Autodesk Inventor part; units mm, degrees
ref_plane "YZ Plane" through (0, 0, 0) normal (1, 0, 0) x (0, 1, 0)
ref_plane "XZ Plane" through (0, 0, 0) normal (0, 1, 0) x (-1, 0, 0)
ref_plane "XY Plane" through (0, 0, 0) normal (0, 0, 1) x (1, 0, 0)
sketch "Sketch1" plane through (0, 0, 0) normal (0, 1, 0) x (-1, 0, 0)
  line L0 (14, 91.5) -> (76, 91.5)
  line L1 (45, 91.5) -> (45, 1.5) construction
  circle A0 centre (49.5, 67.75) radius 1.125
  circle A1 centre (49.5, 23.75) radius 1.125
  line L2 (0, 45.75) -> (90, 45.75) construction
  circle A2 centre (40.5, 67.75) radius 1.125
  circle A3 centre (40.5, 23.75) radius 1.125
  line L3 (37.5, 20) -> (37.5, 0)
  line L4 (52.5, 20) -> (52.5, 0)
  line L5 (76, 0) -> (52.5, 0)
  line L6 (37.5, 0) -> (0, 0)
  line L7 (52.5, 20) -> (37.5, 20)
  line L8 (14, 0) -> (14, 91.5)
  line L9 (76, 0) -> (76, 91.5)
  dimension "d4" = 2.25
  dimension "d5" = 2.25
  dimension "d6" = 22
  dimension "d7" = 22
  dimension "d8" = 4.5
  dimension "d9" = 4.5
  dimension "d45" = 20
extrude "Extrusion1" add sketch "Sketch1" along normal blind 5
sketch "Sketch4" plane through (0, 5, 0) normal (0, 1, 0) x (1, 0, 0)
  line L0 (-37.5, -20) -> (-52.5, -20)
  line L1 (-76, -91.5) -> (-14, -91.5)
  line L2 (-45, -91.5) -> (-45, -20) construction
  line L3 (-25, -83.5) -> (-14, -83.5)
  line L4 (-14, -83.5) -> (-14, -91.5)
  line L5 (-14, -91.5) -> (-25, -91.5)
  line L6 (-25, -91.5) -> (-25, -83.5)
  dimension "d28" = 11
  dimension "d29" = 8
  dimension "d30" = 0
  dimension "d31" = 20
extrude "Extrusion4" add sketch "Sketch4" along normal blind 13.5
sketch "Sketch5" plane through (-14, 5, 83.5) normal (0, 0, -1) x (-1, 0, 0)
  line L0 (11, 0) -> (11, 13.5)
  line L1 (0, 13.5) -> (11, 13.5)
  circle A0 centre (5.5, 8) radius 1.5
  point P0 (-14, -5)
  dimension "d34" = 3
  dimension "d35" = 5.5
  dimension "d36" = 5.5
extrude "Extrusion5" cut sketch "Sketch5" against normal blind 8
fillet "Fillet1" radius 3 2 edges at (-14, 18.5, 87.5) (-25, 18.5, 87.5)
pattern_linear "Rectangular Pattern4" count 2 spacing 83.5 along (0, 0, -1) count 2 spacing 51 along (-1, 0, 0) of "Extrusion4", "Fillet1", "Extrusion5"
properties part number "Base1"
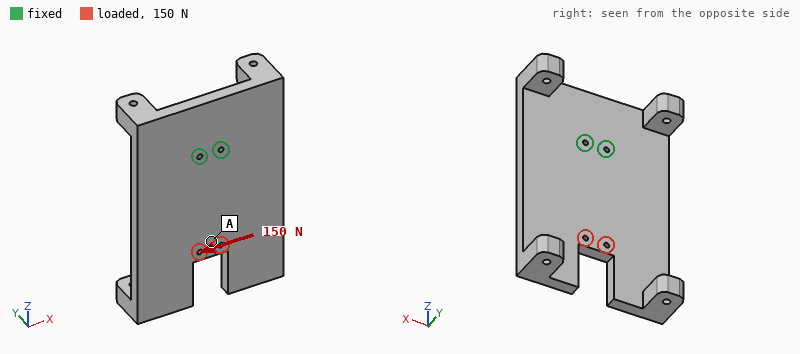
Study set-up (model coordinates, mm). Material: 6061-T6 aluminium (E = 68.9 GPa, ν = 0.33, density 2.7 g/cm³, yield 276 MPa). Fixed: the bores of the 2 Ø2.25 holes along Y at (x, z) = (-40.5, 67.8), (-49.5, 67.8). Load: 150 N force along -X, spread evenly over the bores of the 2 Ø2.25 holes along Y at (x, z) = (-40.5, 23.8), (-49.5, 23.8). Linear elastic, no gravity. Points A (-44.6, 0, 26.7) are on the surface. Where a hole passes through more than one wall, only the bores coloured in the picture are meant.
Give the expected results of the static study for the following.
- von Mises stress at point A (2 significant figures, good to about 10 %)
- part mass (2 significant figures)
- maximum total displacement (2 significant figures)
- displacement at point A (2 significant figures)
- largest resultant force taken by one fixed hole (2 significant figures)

1.8 MPa
84 g
21 µm
12 µm
630 N
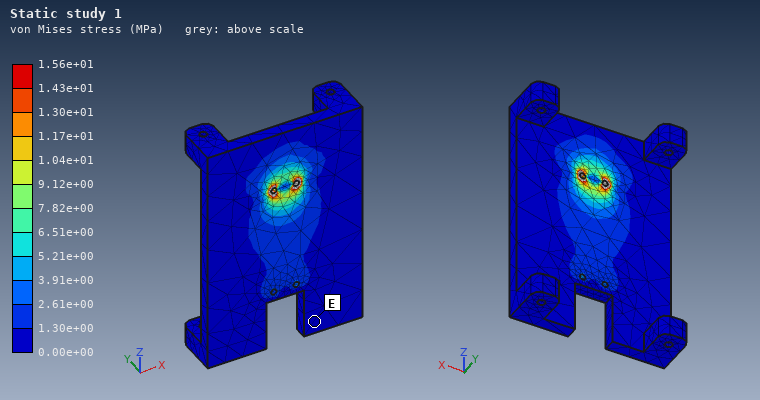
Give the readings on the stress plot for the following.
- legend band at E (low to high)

0.00e+00 to 1.30e+00 MPa
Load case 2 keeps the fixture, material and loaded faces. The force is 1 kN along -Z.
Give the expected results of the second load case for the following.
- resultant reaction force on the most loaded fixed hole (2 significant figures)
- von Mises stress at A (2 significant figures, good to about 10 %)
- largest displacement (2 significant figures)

500 N
6.9 MPa
5.5 µm
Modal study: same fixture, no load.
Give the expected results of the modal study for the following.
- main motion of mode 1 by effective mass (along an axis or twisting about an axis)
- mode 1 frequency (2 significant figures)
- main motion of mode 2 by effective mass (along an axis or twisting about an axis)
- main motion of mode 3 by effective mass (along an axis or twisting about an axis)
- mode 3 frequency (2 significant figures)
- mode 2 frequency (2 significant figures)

along Y
700 Hz
twisting about Z
along X
2100 Hz
1300 Hz
